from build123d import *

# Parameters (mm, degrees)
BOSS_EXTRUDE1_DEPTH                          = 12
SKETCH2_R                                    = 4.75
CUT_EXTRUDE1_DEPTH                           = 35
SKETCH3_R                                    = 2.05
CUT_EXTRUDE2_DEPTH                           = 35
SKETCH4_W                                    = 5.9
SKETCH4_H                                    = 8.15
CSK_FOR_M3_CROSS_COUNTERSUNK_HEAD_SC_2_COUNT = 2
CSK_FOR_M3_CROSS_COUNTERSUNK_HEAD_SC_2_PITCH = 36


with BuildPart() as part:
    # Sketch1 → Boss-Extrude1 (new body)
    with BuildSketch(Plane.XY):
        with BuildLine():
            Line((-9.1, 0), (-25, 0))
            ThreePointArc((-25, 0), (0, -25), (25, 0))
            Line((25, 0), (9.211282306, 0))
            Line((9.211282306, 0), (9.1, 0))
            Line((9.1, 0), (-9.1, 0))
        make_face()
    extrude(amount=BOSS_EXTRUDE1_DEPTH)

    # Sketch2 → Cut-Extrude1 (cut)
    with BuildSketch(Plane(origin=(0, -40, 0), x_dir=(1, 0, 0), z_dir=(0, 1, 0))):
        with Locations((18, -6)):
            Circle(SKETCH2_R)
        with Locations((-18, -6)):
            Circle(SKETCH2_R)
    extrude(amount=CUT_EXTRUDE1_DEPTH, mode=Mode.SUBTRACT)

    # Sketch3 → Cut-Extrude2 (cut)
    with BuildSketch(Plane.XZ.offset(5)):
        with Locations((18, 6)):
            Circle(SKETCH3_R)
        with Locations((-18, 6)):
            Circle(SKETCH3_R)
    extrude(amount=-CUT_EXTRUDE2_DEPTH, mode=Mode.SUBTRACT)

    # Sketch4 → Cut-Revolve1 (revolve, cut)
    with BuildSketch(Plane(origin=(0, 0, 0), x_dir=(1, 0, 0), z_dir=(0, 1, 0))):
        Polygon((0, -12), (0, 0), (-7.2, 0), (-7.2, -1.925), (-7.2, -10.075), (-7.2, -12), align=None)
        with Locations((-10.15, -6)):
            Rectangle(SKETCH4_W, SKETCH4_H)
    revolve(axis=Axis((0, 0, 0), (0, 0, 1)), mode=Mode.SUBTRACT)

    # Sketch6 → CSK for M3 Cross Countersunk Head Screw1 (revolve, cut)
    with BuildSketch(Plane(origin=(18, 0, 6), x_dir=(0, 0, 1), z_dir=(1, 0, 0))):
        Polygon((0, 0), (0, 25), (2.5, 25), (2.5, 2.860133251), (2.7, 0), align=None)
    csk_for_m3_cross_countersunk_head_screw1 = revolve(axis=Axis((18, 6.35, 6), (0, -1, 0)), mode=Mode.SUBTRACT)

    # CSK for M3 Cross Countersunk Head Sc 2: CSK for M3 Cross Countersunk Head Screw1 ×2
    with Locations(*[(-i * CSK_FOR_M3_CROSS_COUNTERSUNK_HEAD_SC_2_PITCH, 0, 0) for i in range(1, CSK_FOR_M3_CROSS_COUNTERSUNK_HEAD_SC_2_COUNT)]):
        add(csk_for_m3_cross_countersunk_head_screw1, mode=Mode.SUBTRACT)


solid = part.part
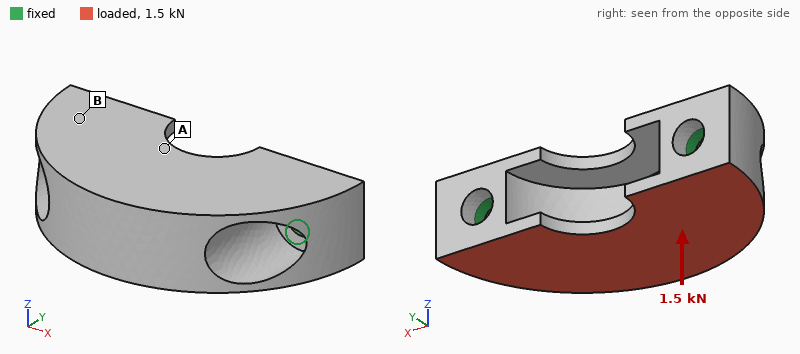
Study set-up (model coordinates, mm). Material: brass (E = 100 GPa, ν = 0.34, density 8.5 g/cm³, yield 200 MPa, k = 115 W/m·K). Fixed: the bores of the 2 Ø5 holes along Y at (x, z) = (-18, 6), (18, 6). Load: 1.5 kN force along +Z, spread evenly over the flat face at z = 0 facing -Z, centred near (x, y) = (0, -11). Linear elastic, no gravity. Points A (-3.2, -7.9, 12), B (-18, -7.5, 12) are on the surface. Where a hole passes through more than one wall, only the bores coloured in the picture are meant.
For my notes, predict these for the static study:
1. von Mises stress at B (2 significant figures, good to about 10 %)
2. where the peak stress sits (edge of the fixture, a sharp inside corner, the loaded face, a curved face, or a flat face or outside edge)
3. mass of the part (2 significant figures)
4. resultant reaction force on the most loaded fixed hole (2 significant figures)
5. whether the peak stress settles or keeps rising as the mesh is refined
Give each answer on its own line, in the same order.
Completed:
36 MPa
edge of the fixture
63 g
750 N
keeps rising
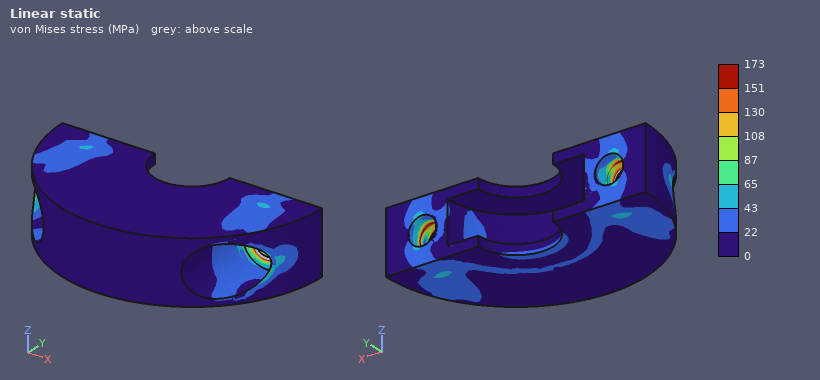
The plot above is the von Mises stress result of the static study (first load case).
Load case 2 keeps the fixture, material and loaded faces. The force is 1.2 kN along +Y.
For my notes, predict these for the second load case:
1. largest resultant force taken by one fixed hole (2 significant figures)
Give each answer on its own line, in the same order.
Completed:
640 N
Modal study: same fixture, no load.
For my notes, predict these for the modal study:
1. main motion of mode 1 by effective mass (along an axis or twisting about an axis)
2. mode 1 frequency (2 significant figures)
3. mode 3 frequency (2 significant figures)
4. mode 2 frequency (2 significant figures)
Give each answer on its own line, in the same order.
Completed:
along Z
4100 Hz
14 kHz
14 kHz
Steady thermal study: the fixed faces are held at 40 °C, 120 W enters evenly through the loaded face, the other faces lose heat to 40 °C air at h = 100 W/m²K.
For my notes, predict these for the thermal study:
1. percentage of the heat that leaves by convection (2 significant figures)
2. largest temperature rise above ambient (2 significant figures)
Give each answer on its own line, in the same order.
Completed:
12 %
73 K
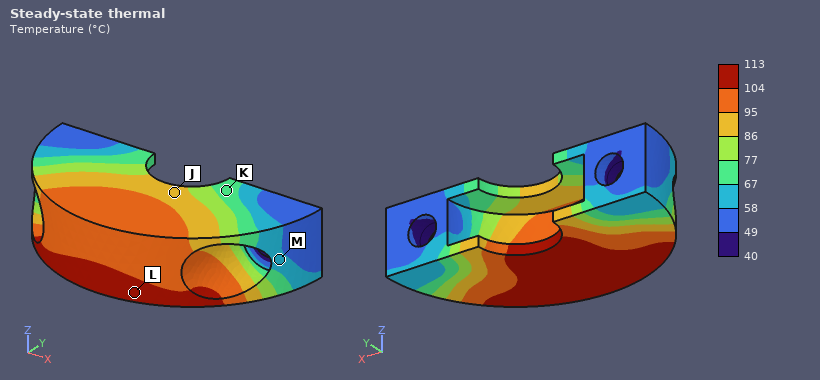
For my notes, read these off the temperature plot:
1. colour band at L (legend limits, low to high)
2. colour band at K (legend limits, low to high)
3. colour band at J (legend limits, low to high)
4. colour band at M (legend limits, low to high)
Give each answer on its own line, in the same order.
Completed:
104 to 113 °C
67 to 77 °C
86 to 95 °C
58 to 67 °C
